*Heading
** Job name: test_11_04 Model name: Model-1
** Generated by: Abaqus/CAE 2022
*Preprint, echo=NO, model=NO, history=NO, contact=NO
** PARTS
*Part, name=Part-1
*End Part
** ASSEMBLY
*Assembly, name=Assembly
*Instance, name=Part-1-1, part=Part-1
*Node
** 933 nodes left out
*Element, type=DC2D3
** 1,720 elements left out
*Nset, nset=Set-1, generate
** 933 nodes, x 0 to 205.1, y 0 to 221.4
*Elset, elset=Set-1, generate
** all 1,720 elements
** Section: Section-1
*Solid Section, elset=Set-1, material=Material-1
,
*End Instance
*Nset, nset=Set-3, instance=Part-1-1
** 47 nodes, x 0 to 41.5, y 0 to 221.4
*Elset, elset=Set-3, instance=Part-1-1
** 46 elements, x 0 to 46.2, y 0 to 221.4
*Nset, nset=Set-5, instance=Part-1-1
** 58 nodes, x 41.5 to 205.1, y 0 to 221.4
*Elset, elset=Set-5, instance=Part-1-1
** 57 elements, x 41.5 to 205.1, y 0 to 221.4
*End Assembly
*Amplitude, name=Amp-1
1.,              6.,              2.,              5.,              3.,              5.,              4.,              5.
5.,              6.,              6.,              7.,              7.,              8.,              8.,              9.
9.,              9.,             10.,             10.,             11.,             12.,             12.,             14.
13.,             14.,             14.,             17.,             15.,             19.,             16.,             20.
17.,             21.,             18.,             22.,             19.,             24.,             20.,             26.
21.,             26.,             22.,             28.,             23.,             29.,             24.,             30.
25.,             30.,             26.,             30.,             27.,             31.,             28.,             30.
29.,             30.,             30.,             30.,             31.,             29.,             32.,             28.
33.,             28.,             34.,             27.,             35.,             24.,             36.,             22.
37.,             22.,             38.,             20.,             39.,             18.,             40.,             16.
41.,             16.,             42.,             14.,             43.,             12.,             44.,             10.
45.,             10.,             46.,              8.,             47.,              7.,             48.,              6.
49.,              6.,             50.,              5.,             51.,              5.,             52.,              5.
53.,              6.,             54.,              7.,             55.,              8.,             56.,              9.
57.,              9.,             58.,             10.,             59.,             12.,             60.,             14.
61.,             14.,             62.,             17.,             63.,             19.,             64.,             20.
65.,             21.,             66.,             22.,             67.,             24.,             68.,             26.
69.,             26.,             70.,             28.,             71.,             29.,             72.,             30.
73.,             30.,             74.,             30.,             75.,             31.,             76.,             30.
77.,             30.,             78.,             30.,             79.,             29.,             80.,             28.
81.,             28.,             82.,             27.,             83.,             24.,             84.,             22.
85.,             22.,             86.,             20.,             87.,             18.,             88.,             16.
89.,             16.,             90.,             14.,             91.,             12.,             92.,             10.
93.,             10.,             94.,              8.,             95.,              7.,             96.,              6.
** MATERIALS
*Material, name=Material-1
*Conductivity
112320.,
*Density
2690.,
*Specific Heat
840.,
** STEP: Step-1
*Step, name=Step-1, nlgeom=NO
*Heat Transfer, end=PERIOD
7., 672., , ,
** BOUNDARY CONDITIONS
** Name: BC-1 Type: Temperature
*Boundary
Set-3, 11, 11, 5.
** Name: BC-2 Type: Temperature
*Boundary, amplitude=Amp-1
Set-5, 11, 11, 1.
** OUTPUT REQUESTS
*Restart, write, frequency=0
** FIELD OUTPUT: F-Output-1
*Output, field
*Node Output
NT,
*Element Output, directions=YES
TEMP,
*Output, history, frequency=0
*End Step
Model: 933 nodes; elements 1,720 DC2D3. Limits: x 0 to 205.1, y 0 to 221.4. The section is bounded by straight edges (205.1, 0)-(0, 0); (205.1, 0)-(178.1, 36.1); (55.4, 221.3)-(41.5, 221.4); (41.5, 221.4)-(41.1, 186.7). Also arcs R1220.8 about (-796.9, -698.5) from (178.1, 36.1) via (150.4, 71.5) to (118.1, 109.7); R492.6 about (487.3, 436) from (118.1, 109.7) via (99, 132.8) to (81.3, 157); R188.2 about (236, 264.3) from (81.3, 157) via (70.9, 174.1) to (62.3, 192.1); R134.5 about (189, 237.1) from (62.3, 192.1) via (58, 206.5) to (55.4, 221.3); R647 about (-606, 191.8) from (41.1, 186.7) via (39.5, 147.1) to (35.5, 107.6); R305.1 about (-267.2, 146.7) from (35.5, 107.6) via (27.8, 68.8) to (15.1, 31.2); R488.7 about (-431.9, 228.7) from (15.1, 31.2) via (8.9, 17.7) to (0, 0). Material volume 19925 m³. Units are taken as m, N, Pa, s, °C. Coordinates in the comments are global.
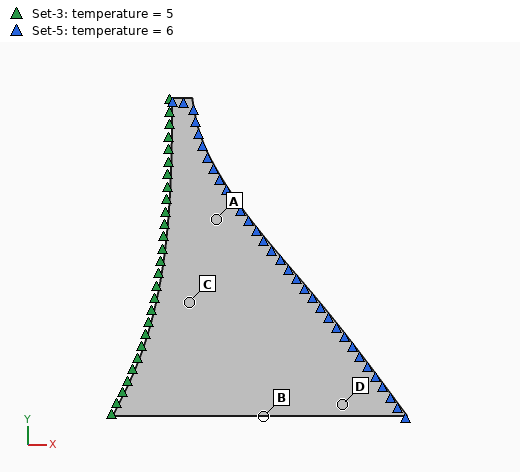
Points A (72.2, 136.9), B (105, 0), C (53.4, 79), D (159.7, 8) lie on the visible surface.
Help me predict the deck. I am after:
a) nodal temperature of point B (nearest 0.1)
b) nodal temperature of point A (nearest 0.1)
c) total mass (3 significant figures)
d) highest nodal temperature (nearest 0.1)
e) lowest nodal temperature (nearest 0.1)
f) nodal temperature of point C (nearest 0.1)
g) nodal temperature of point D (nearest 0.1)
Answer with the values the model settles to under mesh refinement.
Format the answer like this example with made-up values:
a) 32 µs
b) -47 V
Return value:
a) 0.0 °C
b) 0.2 °C
c) 5.36e+07 kg
d) 6.0 °C
e) 0.0 °C
f) 0.0 °C
g) 0.0 °C
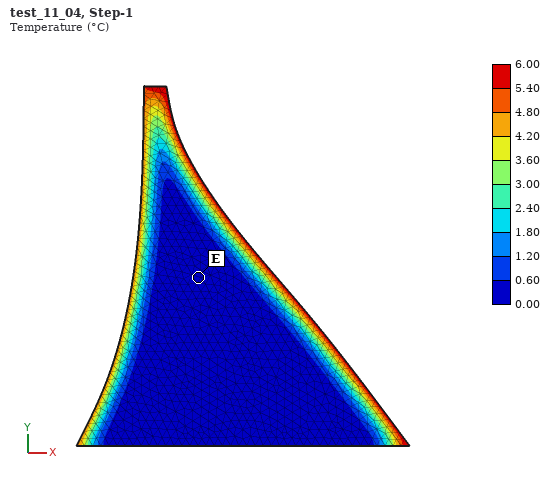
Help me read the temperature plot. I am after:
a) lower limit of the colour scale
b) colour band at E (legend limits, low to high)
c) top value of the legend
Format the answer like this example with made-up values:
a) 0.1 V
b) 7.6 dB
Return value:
a) 0.00 °C
b) 0.00 to 0.60 °C
c) 6.00 °C
